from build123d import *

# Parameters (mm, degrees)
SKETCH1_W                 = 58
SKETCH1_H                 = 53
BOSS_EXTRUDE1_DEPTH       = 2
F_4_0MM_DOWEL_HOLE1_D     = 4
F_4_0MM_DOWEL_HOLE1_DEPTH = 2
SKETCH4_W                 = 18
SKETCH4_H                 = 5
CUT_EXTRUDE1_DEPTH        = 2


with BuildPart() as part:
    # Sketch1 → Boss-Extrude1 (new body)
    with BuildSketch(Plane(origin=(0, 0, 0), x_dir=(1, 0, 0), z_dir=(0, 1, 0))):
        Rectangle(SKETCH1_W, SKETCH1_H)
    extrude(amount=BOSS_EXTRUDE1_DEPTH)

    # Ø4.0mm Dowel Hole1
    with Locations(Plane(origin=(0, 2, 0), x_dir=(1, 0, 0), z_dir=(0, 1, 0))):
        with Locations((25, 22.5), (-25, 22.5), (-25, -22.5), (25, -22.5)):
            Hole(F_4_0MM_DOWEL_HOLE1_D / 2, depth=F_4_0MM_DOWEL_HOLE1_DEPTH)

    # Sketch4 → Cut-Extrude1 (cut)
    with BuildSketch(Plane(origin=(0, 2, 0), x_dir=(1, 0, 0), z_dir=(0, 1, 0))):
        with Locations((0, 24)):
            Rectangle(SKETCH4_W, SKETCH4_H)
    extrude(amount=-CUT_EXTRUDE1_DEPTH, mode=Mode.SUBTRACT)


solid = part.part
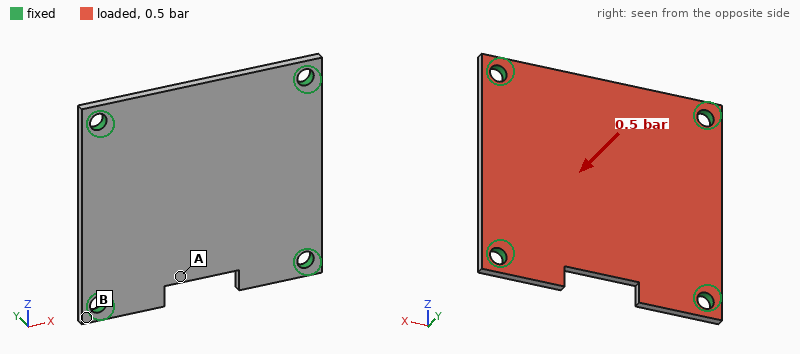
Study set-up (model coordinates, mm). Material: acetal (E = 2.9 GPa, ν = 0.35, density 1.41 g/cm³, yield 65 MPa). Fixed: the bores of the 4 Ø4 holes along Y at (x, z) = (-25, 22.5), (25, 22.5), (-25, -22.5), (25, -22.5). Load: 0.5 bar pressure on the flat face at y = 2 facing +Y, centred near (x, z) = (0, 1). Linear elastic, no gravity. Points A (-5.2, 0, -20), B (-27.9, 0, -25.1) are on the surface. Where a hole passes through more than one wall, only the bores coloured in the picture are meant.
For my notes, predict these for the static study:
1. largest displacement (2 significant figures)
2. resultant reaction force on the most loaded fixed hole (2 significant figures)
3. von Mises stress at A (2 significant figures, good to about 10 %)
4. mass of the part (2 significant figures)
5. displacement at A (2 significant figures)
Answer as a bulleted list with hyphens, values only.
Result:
- 0.79 mm
- 38 N
- 9.2 MPa
- 8.3 g
- 0.51 mm
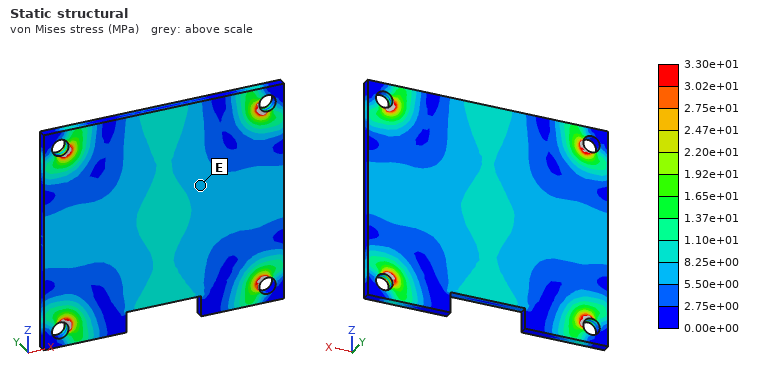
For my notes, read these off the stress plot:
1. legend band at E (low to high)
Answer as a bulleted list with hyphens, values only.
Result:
- 5.50e+00 to 8.25e+00 MPa
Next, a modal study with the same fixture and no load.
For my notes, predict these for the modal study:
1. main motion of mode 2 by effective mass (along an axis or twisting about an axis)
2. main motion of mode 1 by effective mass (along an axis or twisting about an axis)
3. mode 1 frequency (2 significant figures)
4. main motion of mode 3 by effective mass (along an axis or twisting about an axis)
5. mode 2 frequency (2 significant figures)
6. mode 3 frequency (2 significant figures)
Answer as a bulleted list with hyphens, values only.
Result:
- twisting about X
- along Y
- 910 Hz
- twisting about Z
- 1500 Hz
- 1700 Hz
